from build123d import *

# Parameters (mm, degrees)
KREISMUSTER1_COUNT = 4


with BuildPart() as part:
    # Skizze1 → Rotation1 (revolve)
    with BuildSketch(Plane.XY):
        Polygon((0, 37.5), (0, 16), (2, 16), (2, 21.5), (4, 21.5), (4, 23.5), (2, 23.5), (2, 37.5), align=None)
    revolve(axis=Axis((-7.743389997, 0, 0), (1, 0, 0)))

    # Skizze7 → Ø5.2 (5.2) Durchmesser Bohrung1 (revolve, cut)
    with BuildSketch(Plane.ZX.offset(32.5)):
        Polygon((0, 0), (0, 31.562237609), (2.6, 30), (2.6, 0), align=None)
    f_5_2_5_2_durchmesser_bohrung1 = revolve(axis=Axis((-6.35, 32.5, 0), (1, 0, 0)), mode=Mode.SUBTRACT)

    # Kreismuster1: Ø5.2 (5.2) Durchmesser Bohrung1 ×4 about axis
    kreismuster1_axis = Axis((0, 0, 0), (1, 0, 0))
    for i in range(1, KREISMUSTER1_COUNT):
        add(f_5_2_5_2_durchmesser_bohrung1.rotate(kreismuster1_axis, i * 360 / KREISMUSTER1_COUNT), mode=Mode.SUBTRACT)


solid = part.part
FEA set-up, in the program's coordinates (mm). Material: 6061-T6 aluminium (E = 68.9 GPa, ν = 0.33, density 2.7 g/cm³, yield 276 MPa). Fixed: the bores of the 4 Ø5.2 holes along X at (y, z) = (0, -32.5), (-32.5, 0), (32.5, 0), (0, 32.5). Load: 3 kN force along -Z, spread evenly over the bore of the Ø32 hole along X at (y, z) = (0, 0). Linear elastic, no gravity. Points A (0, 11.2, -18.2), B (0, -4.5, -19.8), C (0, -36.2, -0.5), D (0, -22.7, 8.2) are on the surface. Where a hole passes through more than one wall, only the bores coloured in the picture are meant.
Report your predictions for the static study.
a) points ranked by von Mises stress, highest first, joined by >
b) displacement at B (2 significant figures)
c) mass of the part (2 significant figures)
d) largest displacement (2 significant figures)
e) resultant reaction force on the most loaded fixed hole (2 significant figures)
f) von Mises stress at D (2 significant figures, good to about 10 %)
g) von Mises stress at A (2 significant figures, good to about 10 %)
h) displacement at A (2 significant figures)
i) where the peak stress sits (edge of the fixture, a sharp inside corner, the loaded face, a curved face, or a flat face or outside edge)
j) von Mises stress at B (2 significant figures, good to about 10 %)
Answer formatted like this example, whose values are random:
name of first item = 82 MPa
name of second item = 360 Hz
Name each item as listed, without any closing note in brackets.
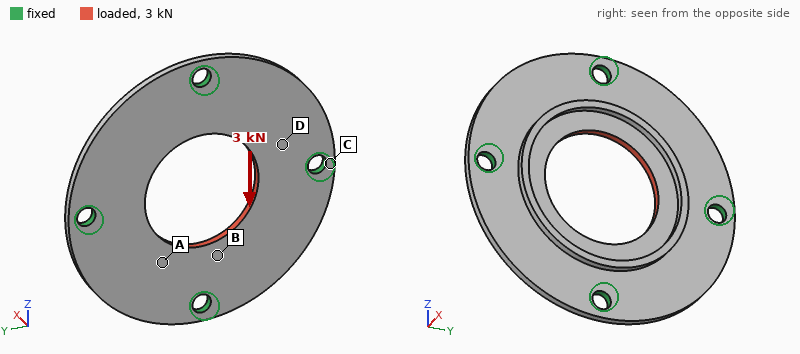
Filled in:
points ranked by von Mises stress, highest first, joined by > = B > A > D > C
displacement at B = 5.3 µm
mass of the part = 21 g
largest displacement = 9.4 µm
resultant reaction force on the most loaded fixed hole = 840 N
von Mises stress at D = 10 MPa
von Mises stress at A = 18 MPa
displacement at A = 7.1 µm
where the peak stress sits = edge of the fixture
von Mises stress at B = 25 MPa
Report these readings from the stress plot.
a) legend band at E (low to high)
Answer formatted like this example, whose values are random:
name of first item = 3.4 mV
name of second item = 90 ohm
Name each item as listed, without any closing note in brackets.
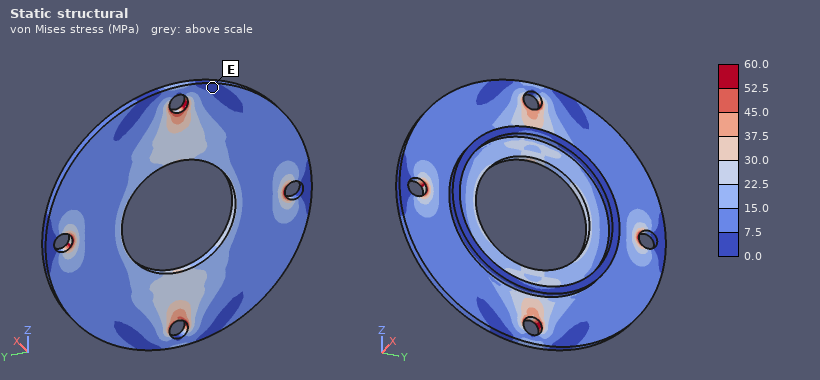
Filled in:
legend band at E = 0.0 to 7.5 MPa
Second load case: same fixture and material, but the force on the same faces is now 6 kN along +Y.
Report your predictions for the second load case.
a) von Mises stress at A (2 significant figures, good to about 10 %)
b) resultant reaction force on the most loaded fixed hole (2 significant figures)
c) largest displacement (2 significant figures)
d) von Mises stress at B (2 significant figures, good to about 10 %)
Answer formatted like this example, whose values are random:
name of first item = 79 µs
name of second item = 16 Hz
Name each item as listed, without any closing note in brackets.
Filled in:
von Mises stress at A = 21 MPa
resultant reaction force on the most loaded fixed hole = 1.7 kN
largest displacement = 19 µm
von Mises stress at B = 20 MPa
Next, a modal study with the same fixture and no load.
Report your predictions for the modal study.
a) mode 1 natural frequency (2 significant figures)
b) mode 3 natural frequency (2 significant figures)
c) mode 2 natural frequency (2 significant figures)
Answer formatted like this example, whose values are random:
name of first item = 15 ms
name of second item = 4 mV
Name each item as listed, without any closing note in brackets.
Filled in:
mode 1 natural frequency = 4700 Hz
mode 3 natural frequency = 5100 Hz
mode 2 natural frequency = 5100 Hz
